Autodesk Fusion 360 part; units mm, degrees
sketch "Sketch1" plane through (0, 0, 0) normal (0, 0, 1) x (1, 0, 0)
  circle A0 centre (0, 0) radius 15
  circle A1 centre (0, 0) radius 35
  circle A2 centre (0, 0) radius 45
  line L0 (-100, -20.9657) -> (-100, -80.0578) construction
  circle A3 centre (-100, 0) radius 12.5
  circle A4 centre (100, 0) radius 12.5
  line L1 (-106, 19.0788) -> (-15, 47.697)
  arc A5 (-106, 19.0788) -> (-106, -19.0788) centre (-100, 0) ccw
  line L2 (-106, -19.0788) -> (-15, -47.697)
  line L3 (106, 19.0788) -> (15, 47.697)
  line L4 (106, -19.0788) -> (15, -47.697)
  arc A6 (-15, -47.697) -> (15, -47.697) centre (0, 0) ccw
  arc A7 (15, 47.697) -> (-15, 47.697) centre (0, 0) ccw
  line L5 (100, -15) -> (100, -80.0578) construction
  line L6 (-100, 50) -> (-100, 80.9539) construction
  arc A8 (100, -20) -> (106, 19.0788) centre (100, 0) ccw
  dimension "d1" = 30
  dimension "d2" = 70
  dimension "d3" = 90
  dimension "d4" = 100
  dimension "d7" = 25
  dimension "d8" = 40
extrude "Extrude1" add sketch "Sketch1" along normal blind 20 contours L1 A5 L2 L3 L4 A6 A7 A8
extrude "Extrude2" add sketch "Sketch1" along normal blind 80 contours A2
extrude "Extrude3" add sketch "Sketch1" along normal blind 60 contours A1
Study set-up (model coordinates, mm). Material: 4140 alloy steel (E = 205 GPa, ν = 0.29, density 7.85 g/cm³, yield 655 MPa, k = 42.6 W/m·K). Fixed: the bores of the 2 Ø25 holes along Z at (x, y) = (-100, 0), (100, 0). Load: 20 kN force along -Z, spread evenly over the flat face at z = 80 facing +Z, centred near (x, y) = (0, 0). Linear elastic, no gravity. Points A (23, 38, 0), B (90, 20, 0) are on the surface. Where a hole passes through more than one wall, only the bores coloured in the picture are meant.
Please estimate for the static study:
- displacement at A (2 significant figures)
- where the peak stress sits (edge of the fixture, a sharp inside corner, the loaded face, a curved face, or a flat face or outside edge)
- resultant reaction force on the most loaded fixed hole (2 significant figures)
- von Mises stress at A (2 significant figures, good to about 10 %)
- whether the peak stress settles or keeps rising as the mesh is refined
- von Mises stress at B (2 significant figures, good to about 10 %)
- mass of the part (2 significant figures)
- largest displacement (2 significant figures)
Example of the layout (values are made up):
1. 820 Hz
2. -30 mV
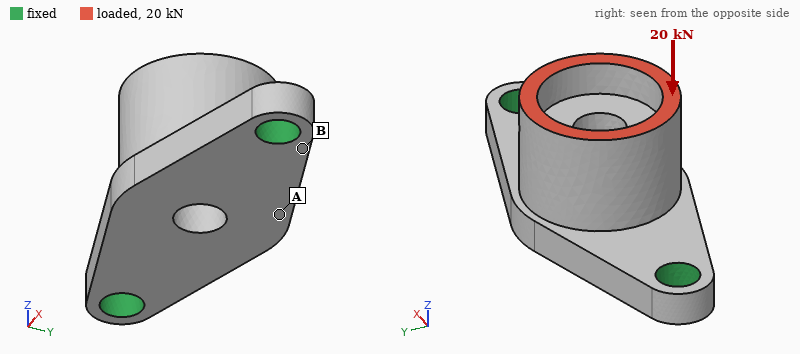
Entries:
1. 31 µm
2. edge of the fixture
3. 11 kN
4. 18 MPa
5. keeps rising
6. 44 MPa
7. 4.4 kg
8. 34 µm
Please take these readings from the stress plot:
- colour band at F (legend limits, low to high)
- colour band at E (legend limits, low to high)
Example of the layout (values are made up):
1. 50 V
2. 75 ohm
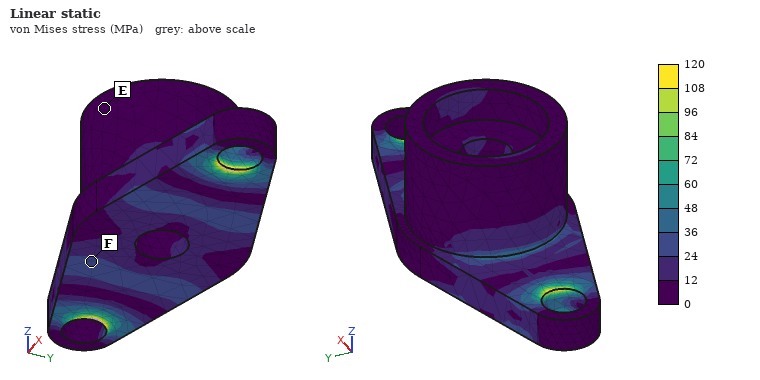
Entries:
1. 24 to 36 MPa
2. 0 to 12 MPa
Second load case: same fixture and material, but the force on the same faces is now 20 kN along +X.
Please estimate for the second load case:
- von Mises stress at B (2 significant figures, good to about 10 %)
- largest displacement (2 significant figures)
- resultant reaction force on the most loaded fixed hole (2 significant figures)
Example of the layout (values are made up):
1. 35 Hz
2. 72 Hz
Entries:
1. 34 MPa
2. 52 µm
3. 14 kN
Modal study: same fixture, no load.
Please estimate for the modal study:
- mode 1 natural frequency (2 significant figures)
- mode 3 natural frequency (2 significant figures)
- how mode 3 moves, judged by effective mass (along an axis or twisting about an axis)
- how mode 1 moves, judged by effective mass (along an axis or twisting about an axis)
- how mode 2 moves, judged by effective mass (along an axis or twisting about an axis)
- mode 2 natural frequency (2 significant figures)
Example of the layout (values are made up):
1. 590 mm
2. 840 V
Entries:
1. 1400 Hz
2. 3600 Hz
3. along X
4. along Y
5. along Z
6. 2200 Hz
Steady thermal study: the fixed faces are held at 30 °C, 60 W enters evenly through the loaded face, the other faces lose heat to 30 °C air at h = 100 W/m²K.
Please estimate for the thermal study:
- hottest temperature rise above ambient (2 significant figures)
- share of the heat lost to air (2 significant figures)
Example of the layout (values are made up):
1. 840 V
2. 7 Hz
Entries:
1. 23 K
2. 84 %
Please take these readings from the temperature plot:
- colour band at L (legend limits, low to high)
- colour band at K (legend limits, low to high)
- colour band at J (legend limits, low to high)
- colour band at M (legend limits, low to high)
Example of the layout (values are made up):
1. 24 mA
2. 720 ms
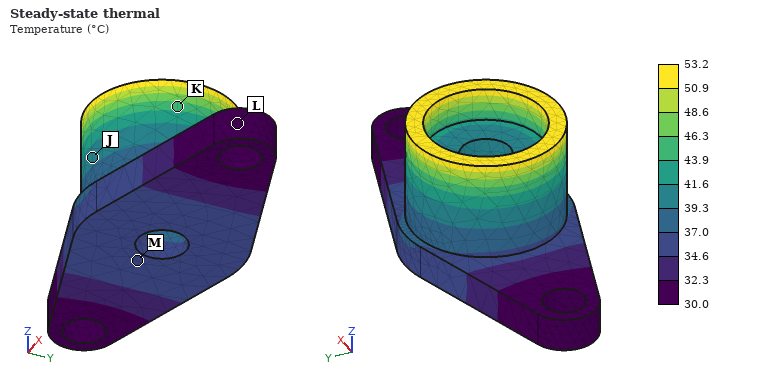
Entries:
1. 30.0 to 32.3 °C
2. 43.9 to 46.3 °C
3. 39.3 to 41.6 °C
4. 34.6 to 37.0 °C
